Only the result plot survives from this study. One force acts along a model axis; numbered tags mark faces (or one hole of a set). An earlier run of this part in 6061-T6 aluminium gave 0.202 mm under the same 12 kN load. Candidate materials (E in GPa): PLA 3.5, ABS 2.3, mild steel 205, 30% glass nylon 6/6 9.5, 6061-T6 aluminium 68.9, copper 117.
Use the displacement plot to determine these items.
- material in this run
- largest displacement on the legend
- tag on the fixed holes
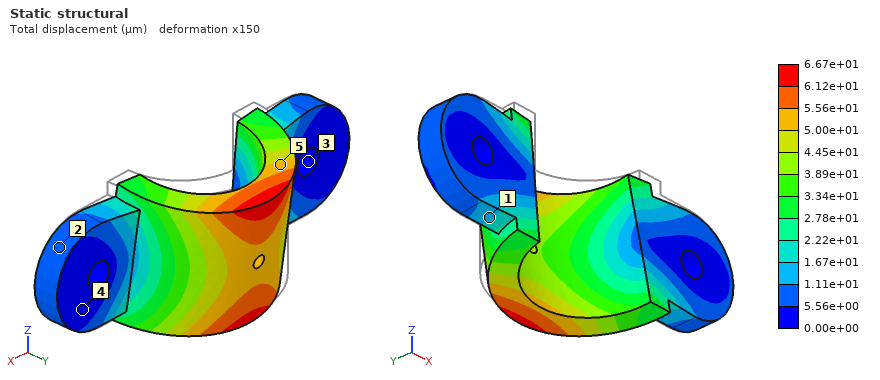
mild steel
6.67e+01 µm
3
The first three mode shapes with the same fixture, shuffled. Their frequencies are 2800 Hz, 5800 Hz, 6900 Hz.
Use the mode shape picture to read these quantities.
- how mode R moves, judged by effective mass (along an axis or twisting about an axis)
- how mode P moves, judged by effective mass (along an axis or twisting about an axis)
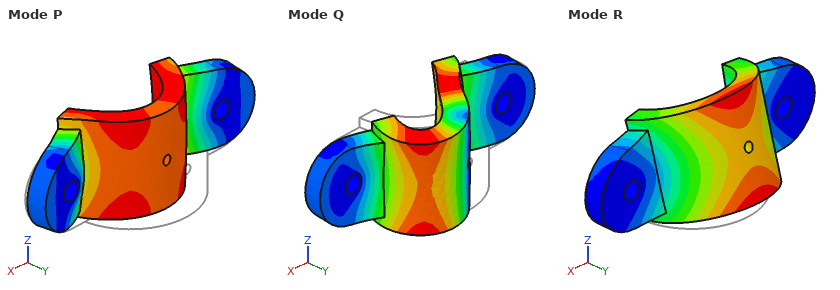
along Z
along Y
